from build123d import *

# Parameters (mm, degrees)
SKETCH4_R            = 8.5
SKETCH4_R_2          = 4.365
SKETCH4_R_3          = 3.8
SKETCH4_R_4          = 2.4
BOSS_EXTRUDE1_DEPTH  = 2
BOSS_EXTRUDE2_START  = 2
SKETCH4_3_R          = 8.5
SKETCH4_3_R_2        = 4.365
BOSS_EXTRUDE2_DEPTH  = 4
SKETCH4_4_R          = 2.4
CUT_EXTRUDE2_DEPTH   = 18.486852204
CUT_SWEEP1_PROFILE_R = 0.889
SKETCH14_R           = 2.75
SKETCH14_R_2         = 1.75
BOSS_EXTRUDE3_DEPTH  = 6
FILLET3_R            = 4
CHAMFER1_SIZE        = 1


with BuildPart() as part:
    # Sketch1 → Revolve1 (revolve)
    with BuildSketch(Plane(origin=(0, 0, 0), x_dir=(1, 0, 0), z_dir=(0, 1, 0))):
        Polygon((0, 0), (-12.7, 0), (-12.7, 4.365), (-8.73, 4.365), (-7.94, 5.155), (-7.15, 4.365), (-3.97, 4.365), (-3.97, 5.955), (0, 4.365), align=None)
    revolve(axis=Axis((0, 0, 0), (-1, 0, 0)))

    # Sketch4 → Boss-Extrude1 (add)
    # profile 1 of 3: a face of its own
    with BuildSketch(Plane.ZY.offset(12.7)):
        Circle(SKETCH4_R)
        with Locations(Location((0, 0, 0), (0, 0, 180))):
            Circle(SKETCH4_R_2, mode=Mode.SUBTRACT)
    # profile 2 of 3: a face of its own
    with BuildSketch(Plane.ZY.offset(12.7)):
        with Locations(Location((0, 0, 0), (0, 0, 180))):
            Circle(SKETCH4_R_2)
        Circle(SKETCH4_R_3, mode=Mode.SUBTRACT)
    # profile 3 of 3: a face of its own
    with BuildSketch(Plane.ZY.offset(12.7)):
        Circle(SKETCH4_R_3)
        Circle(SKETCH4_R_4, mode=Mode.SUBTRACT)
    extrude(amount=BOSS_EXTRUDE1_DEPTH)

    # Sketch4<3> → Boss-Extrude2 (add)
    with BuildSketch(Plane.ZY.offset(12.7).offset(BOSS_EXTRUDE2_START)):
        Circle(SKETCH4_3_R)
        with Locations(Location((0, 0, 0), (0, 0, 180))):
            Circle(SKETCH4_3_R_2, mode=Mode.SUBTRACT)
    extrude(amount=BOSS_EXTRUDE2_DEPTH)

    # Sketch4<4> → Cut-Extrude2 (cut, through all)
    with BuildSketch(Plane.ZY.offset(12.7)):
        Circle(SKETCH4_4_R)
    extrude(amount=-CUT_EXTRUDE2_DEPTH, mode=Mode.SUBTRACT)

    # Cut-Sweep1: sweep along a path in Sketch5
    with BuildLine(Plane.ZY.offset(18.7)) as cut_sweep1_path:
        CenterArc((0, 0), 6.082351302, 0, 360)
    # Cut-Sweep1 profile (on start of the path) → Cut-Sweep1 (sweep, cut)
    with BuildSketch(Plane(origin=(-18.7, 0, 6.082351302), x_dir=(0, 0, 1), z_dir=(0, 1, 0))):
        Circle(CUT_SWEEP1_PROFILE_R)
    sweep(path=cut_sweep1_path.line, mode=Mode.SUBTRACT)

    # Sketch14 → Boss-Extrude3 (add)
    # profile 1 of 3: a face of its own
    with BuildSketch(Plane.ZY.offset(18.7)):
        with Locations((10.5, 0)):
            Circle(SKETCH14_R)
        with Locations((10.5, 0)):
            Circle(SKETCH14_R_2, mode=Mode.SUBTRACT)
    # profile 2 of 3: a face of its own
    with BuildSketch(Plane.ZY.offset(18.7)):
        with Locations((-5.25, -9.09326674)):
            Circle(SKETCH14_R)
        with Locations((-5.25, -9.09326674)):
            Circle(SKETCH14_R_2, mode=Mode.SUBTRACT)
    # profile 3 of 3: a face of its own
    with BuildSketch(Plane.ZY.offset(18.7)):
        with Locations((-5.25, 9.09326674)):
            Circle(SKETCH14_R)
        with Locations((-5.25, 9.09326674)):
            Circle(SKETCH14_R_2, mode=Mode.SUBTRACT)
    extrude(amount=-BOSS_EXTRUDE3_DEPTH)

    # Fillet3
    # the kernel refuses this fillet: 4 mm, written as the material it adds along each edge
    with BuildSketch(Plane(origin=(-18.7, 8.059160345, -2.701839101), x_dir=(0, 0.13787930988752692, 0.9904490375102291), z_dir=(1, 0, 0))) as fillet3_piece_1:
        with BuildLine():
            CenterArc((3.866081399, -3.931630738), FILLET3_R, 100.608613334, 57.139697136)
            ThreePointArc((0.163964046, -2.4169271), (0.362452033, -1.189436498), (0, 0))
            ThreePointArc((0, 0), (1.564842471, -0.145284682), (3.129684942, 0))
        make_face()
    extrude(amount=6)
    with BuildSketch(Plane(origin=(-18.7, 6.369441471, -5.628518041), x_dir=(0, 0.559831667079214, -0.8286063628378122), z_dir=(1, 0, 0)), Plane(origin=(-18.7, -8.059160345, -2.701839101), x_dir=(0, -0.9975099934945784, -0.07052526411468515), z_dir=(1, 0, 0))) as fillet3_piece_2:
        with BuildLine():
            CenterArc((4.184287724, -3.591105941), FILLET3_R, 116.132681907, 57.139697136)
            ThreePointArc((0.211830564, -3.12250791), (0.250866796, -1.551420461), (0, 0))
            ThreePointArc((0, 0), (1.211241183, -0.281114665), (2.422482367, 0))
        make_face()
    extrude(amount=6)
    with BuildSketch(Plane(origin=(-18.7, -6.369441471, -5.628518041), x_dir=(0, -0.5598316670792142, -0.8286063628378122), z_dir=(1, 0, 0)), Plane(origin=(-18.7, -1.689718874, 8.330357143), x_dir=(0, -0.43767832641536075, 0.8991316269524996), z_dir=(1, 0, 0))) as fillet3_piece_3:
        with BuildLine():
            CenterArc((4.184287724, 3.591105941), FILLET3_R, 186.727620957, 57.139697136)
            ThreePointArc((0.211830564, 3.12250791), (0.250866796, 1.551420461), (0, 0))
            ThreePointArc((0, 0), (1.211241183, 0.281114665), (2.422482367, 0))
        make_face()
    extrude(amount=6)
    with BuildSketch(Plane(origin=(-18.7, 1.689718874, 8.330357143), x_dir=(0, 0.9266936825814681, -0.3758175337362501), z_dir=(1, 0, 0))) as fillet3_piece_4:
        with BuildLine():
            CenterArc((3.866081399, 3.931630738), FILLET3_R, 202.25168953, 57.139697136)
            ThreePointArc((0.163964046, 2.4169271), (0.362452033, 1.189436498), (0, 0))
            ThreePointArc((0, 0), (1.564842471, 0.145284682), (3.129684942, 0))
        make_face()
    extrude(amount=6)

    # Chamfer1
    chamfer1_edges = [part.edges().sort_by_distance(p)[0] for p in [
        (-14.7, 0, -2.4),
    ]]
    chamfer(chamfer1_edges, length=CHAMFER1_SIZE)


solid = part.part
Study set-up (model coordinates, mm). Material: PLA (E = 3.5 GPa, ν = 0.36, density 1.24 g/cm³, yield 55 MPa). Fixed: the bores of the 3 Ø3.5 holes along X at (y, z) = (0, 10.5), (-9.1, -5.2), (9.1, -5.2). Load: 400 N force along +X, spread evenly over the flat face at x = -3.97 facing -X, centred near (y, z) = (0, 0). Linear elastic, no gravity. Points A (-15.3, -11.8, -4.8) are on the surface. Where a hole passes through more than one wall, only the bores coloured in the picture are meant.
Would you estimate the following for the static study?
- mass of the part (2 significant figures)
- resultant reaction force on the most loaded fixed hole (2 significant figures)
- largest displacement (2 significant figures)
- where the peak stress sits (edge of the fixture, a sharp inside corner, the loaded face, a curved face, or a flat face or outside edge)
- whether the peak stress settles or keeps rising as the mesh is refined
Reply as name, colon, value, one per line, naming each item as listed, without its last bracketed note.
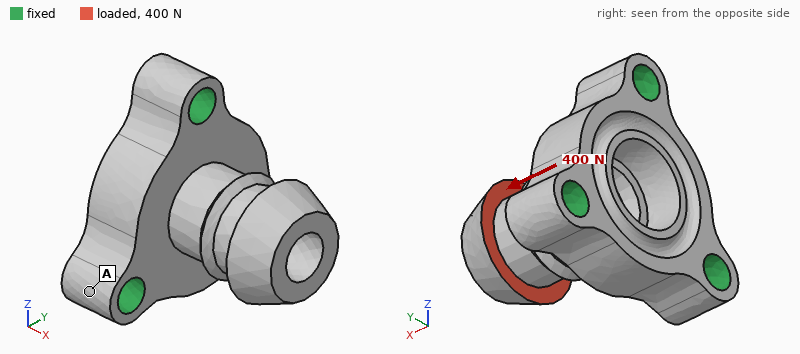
mass of the part: 2.4 g
resultant reaction force on the most loaded fixed hole: 140 N
largest displacement: 70 µm
where the peak stress sits: edge of the fixture
whether the peak stress settles or keeps rising as the mesh is refined: keeps rising
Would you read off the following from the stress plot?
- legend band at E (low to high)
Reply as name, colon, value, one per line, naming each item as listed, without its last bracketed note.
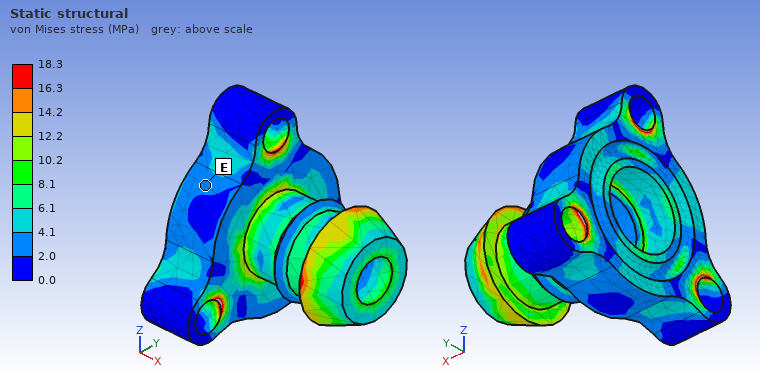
legend band at E: 2.0 to 4.1 MPa
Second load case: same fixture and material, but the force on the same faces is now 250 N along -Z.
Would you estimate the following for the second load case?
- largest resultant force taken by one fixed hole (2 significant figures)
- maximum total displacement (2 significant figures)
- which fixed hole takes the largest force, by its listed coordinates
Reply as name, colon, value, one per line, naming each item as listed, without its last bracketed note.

largest resultant force taken by one fixed hole: 250 N
maximum total displacement: 0.34 mm
which fixed hole takes the largest force, by its listed coordinates: (0, 10.5)
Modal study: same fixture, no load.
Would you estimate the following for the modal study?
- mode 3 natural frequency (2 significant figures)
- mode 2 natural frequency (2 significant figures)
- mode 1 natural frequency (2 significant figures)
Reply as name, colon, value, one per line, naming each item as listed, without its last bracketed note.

mode 3 natural frequency: 14 kHz
mode 2 natural frequency: 6400 Hz
mode 1 natural frequency: 6400 Hz
